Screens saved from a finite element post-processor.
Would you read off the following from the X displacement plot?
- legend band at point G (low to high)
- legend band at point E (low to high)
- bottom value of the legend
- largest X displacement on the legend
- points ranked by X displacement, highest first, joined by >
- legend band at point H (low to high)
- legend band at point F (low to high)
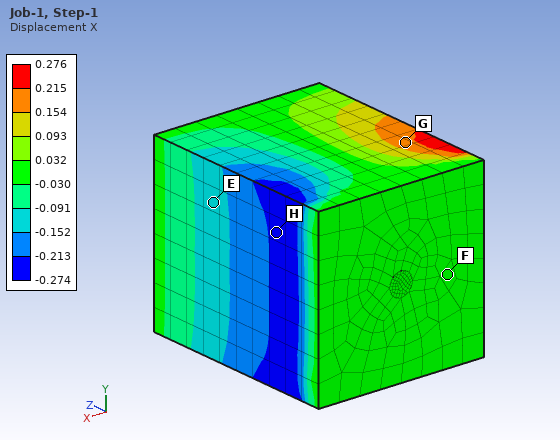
0.154 to 0.215
-0.152 to -0.091
-0.274
0.276
G > F > E > H
-0.274 to -0.213
-0.030 to 0.032
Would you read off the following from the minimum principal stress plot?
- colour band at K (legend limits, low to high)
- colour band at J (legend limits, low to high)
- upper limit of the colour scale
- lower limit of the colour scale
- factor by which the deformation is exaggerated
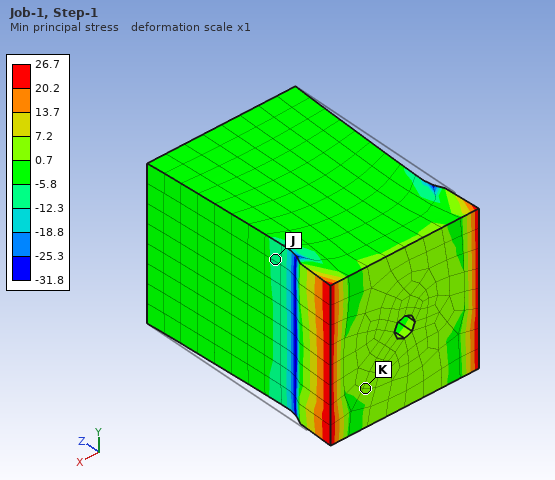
0.7 to 7.2
-12.3 to -5.8
26.7
-31.8
1
